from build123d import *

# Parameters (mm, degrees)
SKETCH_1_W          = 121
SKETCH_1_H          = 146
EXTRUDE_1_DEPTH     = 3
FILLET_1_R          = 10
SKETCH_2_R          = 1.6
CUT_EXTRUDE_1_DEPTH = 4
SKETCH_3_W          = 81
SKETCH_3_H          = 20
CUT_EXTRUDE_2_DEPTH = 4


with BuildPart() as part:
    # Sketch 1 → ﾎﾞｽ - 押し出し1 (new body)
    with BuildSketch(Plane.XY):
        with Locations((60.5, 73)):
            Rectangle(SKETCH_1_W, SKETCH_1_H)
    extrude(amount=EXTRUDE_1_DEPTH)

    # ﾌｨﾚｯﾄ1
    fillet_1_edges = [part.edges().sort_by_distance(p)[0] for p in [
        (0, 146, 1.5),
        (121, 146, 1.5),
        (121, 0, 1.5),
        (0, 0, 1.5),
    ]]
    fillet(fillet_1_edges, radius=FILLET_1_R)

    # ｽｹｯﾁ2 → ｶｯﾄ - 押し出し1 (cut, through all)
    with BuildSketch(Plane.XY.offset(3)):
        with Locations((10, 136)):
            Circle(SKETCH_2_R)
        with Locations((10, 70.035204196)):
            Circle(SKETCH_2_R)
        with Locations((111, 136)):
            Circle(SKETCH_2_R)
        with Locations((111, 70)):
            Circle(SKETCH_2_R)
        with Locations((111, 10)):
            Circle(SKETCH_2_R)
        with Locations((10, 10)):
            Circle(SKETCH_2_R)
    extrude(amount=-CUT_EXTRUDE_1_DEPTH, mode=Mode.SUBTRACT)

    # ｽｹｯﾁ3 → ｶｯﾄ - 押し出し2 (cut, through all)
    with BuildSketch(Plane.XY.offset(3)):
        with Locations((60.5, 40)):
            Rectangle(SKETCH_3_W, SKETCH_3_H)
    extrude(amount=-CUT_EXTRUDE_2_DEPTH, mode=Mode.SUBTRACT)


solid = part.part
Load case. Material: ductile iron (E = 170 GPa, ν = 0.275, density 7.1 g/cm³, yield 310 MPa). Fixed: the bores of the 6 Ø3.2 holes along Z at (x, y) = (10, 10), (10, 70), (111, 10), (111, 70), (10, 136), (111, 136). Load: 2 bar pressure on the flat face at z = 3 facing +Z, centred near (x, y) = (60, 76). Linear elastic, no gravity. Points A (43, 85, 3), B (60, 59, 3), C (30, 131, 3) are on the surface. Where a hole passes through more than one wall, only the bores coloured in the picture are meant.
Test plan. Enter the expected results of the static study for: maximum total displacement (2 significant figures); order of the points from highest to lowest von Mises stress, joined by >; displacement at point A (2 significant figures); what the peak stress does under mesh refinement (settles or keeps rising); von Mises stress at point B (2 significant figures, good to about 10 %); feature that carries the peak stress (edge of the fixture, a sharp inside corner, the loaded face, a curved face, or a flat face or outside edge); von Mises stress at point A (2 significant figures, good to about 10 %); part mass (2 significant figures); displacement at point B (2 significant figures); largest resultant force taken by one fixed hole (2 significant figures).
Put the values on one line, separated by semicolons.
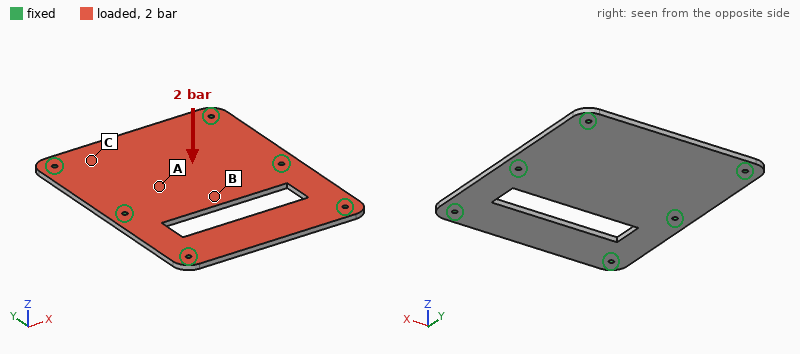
0.22 mm; B > A > C; 0.18 mm; keeps rising; 70 MPa; edge of the fixture; 45 MPa; 340 g; 0.21 mm; 710 N
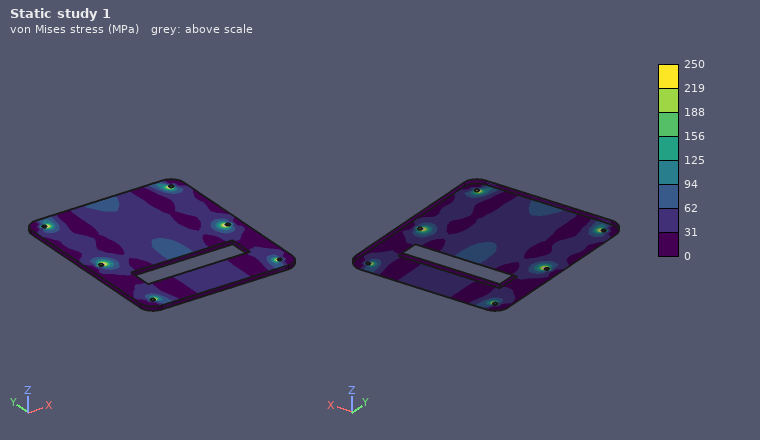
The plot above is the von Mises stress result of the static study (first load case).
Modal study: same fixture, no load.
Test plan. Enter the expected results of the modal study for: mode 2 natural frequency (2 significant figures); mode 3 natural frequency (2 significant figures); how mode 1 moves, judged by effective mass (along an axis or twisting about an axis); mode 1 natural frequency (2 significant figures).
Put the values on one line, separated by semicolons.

1400 Hz; 1700 Hz; along Z; 1200 Hz
